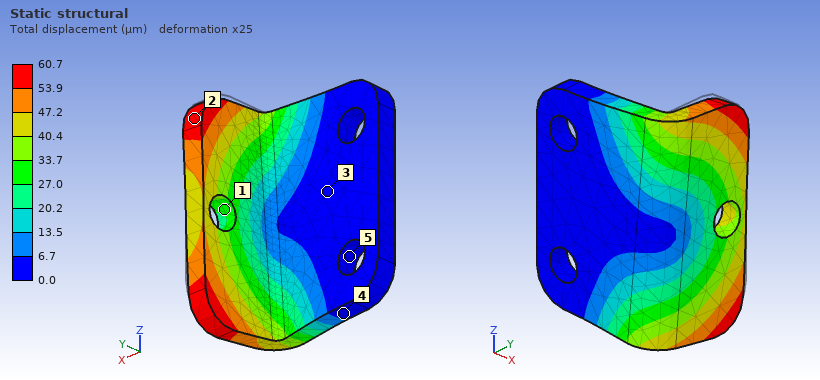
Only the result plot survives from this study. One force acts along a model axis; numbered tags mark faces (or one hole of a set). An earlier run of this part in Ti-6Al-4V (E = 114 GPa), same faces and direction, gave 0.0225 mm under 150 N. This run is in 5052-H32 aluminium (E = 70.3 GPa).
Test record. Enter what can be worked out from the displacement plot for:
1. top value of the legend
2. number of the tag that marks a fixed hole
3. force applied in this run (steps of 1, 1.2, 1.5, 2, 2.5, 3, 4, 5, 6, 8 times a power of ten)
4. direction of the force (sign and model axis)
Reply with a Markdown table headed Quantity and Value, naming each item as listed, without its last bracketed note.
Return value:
| Quantity | Value |
|---|---|
| top value of the legend | 60.7 µm |
| number of the tag that marks a fixed hole | 5 |
| force applied in this run | 250 N |
| direction of the force | -Z |
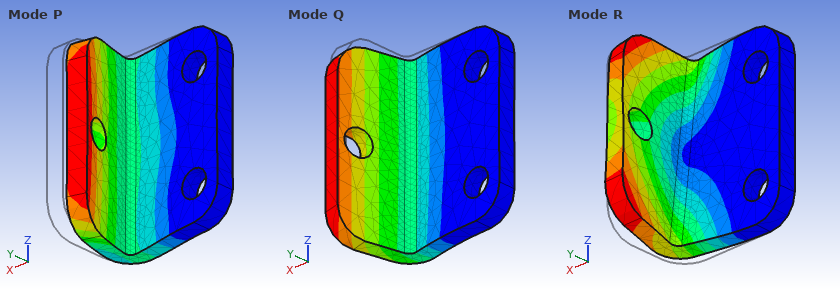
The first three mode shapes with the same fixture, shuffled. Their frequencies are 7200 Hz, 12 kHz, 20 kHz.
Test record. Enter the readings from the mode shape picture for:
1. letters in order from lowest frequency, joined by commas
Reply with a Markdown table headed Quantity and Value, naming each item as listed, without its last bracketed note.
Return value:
| Quantity | Value |
|---|---|
| letters in order from lowest frequency, joined by commas | Q, R, P |
